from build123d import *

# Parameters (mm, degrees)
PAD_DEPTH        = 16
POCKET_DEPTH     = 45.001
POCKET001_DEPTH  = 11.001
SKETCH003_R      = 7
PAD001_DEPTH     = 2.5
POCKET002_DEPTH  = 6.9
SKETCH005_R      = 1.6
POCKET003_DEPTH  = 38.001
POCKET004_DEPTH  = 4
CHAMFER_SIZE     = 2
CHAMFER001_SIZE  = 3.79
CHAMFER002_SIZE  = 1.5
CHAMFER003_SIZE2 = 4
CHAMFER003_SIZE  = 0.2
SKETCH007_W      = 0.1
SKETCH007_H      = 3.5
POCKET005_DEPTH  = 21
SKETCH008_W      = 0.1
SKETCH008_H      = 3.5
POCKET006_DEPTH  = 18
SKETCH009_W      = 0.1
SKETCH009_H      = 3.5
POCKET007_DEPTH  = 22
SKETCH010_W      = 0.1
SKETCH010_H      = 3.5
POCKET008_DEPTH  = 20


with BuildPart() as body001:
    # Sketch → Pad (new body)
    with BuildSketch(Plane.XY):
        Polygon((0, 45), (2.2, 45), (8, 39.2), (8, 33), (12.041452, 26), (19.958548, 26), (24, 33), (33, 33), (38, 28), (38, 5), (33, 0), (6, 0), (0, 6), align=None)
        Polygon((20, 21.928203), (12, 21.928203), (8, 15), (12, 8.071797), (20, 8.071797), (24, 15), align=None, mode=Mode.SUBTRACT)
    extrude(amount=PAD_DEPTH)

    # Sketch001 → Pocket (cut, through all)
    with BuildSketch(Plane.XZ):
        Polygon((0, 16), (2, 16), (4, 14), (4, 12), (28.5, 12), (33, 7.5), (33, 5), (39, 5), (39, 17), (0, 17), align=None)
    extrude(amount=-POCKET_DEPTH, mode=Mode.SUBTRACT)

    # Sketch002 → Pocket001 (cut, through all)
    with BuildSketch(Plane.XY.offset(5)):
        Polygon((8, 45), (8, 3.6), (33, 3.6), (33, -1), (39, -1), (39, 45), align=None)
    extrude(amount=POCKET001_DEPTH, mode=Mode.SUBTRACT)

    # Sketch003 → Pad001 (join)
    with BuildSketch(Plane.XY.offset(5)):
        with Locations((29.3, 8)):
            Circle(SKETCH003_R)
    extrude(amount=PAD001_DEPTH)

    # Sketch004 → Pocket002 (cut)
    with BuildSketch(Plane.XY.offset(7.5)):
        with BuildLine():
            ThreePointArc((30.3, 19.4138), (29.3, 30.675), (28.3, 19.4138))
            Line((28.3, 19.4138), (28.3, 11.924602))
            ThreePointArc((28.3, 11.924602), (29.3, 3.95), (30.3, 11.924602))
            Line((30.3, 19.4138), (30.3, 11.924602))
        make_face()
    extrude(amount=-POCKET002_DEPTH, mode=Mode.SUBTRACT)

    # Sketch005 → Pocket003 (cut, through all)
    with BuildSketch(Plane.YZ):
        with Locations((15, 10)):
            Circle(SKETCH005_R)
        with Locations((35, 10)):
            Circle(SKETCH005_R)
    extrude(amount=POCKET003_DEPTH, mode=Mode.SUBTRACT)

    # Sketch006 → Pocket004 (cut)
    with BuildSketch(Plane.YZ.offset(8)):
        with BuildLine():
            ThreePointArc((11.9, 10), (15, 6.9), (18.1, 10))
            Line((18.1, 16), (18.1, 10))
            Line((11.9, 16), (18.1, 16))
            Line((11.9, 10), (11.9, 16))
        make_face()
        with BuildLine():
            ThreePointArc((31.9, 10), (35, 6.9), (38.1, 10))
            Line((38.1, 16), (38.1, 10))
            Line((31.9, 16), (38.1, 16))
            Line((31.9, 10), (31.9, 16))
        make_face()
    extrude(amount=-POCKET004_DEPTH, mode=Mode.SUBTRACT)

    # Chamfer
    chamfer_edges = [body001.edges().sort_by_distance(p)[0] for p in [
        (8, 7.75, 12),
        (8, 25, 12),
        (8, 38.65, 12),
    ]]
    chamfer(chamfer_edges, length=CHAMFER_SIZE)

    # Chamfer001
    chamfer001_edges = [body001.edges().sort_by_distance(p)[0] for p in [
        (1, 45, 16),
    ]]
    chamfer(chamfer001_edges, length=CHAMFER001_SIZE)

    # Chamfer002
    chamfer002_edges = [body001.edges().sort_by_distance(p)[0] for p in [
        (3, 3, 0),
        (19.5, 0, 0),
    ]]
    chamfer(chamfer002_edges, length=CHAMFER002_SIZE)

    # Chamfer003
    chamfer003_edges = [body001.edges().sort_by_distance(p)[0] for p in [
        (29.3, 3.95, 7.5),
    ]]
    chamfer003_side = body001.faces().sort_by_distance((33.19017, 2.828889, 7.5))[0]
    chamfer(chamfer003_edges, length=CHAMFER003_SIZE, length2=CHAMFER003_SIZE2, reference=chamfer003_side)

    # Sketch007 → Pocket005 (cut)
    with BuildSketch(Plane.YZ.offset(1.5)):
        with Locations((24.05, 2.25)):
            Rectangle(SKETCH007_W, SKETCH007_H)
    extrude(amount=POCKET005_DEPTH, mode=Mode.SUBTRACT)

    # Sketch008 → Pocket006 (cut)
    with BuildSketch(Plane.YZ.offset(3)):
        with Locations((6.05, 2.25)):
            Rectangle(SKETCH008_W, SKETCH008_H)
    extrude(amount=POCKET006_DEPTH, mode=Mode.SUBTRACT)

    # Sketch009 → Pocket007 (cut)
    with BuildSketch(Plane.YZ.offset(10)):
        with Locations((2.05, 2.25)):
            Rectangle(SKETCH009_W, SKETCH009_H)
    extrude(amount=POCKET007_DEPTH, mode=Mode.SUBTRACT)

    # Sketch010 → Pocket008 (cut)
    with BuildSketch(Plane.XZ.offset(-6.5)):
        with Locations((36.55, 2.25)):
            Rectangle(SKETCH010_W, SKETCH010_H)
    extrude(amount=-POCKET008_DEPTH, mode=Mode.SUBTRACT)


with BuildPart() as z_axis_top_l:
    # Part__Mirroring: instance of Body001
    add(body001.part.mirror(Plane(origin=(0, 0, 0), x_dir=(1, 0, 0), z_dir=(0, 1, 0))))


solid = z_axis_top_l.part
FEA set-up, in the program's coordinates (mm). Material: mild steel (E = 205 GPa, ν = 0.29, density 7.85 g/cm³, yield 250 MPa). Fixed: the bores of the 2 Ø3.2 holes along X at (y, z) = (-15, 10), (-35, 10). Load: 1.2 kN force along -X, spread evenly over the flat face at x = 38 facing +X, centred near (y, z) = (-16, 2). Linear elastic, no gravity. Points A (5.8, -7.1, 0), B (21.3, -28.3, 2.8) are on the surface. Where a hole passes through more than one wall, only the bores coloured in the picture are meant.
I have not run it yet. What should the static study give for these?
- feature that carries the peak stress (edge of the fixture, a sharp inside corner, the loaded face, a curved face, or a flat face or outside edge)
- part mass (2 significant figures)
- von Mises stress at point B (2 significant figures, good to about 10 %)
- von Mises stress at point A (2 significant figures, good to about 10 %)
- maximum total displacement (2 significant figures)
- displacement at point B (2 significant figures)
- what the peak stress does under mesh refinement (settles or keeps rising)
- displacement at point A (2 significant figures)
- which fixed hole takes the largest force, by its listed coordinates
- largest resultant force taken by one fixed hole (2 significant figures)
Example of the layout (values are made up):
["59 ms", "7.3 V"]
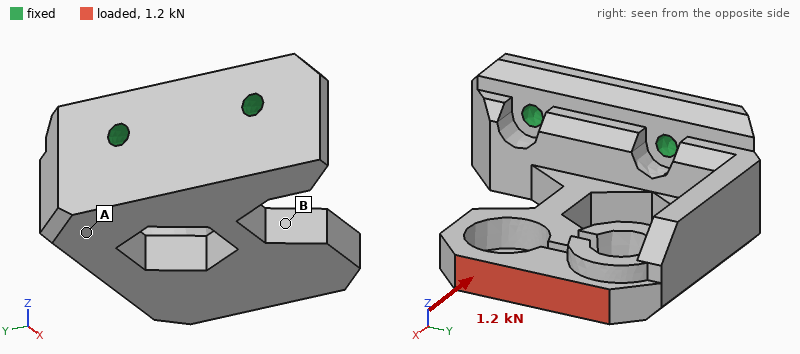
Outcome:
["edge of the fixture", "60 g", "47 MPa", "18 MPa", "35 µm", "20 µm", "keeps rising", "11 µm", "(-15, 10)", "1.0 kN"]
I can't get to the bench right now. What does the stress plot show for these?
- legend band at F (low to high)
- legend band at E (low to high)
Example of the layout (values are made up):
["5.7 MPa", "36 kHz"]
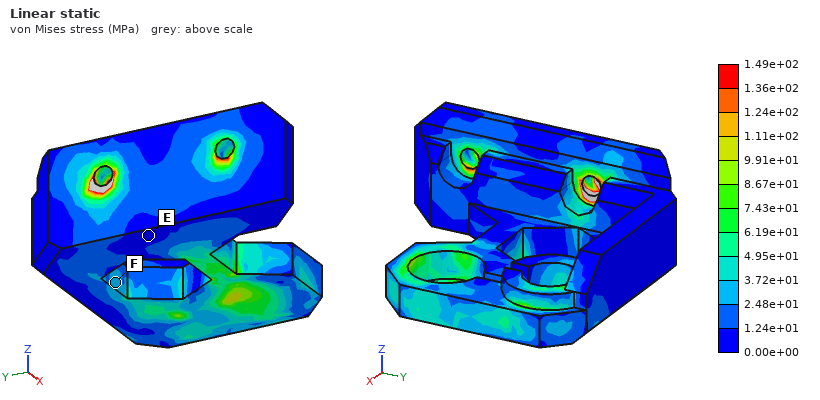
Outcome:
["2.48e+01 to 3.72e+01 MPa", "0.00e+00 to 1.24e+01 MPa"]
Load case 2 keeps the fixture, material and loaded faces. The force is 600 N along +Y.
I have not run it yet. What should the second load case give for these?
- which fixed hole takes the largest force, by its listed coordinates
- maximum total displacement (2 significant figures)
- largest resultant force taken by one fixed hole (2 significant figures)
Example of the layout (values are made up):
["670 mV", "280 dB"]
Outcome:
["(-35, 10)", "55 µm", "1.1 kN"]
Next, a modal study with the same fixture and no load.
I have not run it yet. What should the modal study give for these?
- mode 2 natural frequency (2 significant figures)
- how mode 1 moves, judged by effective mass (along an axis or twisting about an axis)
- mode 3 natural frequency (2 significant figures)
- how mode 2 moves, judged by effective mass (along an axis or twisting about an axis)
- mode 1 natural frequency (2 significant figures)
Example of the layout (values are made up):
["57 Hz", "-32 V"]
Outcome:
["4700 Hz", "along Z", "7100 Hz", "along Y", "2800 Hz"]
